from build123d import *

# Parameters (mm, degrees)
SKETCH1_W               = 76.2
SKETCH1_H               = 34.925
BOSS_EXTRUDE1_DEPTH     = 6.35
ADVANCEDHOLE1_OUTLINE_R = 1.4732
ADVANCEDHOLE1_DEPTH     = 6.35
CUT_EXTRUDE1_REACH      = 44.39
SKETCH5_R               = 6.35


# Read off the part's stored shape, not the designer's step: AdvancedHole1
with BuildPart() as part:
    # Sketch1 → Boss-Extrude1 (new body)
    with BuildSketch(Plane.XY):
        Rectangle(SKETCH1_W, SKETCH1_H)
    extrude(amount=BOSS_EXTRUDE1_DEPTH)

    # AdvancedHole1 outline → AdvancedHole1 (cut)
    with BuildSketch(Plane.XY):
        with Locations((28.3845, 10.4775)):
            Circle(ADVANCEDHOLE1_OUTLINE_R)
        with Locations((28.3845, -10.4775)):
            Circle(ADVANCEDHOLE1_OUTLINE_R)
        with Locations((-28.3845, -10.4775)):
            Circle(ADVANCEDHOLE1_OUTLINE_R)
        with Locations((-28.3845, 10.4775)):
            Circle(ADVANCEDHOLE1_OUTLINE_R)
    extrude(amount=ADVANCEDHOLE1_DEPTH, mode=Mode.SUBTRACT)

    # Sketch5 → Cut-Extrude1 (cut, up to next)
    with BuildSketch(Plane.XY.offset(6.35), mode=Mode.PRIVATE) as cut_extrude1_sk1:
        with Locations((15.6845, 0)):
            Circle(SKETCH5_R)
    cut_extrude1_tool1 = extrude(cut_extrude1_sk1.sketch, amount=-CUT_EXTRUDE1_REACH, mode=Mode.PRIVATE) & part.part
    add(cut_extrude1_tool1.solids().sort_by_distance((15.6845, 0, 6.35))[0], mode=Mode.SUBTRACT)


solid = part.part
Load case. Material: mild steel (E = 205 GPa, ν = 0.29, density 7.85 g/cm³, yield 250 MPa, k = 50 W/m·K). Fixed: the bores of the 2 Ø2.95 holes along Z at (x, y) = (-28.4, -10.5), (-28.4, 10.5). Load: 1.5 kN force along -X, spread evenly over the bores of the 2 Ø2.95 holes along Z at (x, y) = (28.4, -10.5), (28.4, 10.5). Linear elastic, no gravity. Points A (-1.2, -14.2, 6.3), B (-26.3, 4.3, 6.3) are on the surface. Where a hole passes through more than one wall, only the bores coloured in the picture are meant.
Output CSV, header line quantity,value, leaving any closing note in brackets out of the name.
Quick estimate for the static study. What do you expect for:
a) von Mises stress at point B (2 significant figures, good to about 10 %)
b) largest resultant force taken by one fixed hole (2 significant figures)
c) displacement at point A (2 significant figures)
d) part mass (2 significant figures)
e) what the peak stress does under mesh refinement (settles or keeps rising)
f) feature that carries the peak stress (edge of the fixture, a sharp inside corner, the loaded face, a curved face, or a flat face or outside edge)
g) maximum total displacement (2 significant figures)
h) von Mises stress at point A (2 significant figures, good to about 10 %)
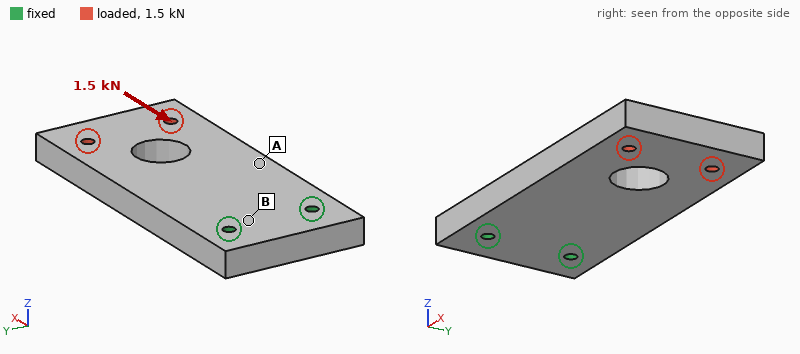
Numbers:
quantity,value
von Mises stress at point B,3.9 MPa
largest resultant force taken by one fixed hole,750 N
displacement at point A,1.1 µm
part mass,120 g
what the peak stress does under mesh refinement,keeps rising
feature that carries the peak stress,edge of the fixture
maximum total displacement,2.7 µm
von Mises stress at point A,8.2 MPa
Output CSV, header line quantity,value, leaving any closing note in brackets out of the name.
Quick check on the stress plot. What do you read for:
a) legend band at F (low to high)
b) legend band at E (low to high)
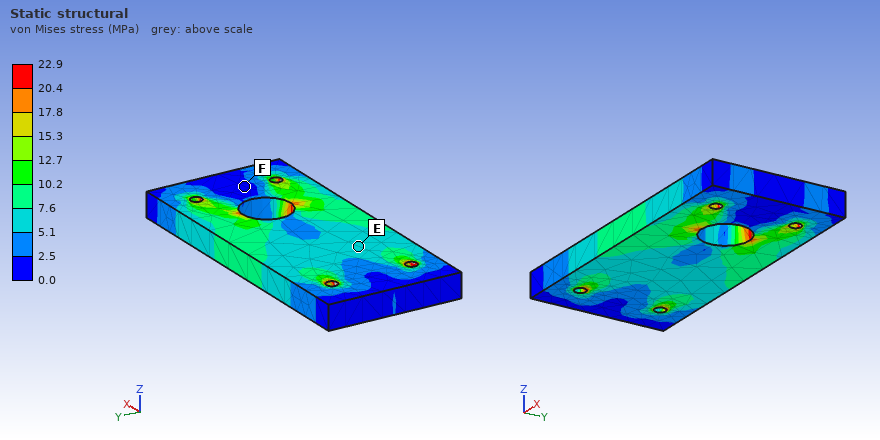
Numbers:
quantity,value
legend band at F,0.0 to 2.5 MPa
legend band at E,5.1 to 7.6 MPa
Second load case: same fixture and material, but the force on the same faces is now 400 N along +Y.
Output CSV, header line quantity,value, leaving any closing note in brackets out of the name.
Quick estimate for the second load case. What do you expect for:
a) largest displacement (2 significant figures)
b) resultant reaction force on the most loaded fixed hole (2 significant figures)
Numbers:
quantity,value
largest displacement,11 µm
resultant reaction force on the most loaded fixed hole,1.0 kN
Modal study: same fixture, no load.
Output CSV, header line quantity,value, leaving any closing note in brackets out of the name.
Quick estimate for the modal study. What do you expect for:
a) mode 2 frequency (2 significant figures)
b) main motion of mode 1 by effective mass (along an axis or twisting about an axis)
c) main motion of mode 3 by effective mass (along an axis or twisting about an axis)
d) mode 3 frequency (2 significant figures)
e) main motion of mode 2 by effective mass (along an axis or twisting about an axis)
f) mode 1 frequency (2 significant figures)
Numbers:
quantity,value
mode 2 frequency,4400 Hz
main motion of mode 1 by effective mass,along Z
main motion of mode 3 by effective mass,along Y
mode 3 frequency,5100 Hz
main motion of mode 2 by effective mass,twisting about X
mode 1 frequency,1200 Hz
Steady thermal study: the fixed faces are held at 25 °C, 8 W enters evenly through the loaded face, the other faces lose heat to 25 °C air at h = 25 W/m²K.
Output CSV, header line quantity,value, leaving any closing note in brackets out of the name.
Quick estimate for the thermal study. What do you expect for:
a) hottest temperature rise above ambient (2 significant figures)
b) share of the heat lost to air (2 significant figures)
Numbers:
quantity,value
hottest temperature rise above ambient,37 K
share of the heat lost to air,35 %
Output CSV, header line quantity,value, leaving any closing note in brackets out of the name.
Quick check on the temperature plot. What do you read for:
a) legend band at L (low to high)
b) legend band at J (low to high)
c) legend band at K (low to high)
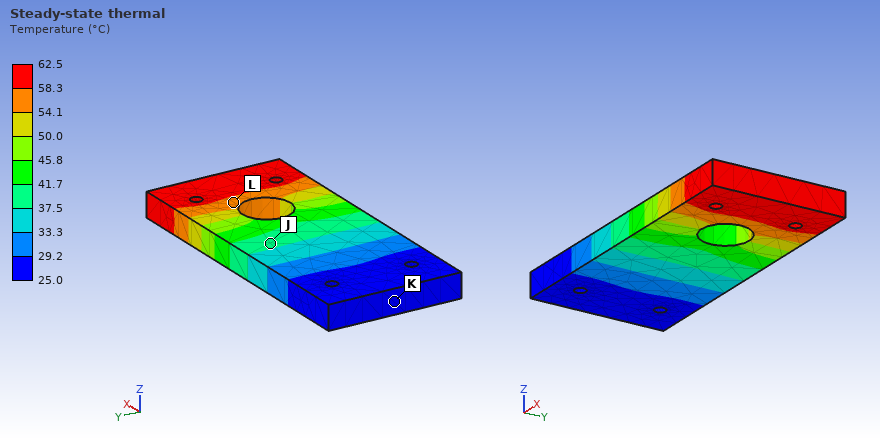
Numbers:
quantity,value
legend band at L,54.1 to 58.3 °C
legend band at J,37.5 to 41.7 °C
legend band at K,25.0 to 29.2 °C
